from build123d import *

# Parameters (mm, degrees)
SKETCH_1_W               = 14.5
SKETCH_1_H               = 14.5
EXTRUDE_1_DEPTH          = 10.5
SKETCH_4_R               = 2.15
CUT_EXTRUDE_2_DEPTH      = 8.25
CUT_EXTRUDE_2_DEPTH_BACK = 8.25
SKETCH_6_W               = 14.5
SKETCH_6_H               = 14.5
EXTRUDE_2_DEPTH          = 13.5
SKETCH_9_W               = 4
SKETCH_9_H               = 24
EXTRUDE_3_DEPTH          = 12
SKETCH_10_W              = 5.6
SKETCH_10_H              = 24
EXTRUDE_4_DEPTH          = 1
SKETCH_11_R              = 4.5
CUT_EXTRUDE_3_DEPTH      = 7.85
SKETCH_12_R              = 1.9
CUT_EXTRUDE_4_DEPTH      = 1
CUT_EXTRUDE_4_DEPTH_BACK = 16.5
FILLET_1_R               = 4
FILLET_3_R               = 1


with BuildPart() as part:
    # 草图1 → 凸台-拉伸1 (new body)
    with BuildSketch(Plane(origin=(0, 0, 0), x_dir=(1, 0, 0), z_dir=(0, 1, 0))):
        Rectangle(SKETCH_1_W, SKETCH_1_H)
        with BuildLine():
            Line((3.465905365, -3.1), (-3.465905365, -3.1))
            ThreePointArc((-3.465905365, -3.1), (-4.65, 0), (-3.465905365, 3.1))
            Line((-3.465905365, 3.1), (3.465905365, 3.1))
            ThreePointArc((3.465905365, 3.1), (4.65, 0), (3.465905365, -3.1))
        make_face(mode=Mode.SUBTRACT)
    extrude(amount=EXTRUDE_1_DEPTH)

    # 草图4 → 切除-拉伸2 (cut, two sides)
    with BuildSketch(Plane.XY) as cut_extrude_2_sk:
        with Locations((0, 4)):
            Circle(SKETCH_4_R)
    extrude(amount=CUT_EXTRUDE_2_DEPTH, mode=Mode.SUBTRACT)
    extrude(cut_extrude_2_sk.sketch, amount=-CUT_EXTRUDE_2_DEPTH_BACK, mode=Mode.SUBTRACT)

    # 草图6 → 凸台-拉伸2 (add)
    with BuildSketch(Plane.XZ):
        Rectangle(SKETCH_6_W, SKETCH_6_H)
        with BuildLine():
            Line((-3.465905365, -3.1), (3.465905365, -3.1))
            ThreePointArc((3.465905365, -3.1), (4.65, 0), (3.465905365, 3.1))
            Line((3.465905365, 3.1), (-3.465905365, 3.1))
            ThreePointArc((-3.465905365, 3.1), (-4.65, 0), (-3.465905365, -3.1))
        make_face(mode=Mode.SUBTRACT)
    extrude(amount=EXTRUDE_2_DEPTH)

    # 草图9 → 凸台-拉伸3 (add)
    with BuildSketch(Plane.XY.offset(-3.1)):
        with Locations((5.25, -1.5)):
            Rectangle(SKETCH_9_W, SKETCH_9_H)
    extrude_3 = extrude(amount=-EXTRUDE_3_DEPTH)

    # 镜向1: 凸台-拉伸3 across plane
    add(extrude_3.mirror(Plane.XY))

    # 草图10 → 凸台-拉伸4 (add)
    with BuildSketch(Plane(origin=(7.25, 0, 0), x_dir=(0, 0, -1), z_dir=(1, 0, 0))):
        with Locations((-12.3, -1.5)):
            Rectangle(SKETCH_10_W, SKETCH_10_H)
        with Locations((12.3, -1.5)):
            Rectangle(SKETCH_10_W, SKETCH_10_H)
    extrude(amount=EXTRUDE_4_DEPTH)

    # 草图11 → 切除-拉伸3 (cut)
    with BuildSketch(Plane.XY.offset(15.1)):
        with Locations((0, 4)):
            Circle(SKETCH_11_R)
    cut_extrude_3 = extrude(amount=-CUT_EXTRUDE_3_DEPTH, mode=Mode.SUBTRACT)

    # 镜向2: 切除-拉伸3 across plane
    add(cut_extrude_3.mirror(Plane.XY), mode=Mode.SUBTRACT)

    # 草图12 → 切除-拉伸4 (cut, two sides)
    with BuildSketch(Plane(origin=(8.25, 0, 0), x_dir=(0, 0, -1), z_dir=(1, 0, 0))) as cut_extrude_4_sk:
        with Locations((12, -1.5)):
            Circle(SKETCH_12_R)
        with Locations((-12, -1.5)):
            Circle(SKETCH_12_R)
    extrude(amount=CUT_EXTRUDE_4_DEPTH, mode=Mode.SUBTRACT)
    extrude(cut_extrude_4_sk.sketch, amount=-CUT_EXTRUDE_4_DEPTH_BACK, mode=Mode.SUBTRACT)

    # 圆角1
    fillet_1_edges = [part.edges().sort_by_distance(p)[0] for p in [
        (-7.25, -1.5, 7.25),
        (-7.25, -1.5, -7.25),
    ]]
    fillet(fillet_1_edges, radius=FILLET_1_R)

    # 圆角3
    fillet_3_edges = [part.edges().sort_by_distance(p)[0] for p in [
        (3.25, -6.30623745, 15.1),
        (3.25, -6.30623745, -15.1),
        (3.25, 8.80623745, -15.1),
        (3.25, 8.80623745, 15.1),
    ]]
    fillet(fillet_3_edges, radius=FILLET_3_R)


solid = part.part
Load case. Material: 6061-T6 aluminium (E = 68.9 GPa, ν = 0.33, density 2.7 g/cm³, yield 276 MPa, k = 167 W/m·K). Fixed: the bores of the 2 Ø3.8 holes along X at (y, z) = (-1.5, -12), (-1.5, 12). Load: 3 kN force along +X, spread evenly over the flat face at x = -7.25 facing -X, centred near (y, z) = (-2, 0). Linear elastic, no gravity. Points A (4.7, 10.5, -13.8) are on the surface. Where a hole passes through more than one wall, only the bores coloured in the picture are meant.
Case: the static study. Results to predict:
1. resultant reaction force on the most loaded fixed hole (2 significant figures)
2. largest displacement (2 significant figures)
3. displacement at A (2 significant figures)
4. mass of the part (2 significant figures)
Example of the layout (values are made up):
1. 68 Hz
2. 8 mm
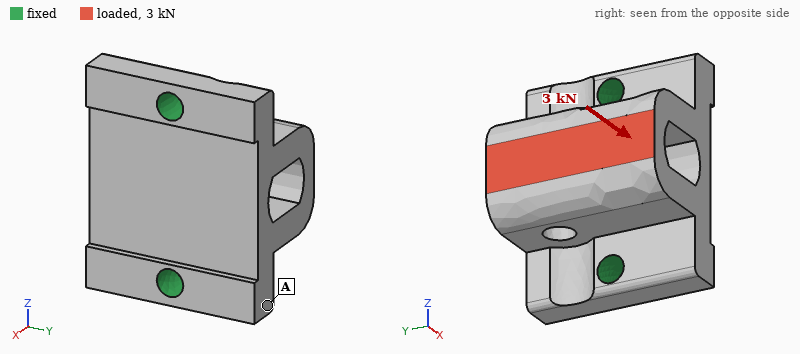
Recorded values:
1. 1.6 kN
2. 24 µm
3. 9.4 µm
4. 14 g
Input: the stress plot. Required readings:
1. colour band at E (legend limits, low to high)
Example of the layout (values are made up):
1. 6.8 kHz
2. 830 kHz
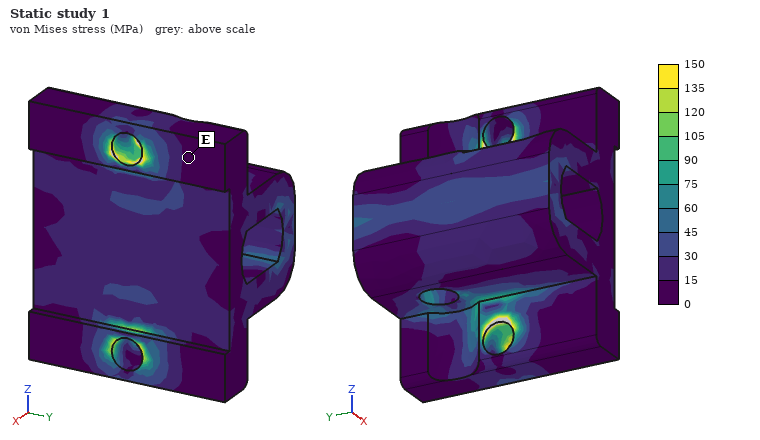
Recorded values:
1. 0 to 15 MPa
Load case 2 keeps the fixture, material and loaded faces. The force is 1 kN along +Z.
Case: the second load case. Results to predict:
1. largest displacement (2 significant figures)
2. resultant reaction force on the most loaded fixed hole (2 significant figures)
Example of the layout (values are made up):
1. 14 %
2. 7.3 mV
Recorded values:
1. 15 µm
2. 810 N
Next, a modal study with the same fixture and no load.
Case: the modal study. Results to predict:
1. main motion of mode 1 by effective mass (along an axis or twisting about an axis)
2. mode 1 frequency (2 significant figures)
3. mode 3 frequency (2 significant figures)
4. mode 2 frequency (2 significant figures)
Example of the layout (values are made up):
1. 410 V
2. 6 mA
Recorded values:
1. along Y
2. 11 kHz
3. 22 kHz
4. 22 kHz
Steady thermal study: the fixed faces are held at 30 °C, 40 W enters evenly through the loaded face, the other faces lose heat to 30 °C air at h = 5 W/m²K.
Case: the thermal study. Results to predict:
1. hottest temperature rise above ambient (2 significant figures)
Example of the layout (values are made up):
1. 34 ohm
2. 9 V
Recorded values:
1. 30 K
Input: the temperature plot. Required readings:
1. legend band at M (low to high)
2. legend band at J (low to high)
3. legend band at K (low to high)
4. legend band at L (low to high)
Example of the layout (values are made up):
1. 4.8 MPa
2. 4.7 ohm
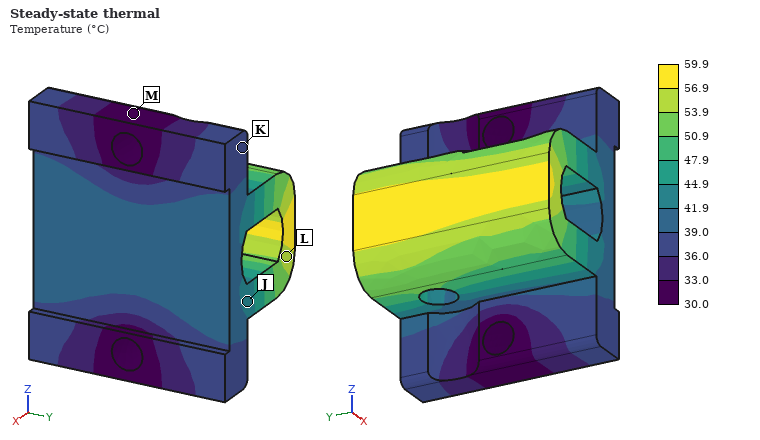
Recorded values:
1. 30.0 to 33.0 °C
2. 41.9 to 44.9 °C
3. 36.0 to 39.0 °C
4. 53.9 to 56.9 °C
